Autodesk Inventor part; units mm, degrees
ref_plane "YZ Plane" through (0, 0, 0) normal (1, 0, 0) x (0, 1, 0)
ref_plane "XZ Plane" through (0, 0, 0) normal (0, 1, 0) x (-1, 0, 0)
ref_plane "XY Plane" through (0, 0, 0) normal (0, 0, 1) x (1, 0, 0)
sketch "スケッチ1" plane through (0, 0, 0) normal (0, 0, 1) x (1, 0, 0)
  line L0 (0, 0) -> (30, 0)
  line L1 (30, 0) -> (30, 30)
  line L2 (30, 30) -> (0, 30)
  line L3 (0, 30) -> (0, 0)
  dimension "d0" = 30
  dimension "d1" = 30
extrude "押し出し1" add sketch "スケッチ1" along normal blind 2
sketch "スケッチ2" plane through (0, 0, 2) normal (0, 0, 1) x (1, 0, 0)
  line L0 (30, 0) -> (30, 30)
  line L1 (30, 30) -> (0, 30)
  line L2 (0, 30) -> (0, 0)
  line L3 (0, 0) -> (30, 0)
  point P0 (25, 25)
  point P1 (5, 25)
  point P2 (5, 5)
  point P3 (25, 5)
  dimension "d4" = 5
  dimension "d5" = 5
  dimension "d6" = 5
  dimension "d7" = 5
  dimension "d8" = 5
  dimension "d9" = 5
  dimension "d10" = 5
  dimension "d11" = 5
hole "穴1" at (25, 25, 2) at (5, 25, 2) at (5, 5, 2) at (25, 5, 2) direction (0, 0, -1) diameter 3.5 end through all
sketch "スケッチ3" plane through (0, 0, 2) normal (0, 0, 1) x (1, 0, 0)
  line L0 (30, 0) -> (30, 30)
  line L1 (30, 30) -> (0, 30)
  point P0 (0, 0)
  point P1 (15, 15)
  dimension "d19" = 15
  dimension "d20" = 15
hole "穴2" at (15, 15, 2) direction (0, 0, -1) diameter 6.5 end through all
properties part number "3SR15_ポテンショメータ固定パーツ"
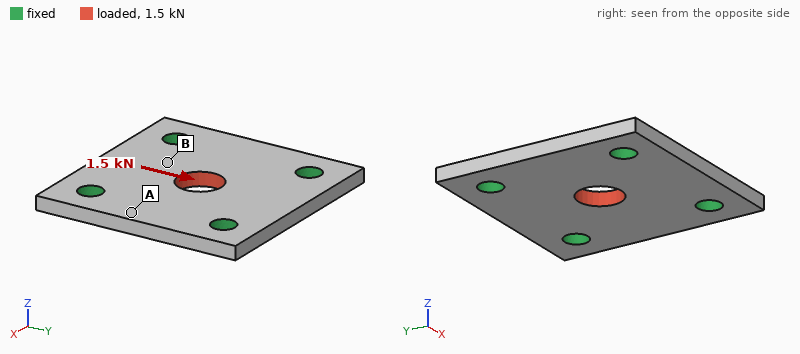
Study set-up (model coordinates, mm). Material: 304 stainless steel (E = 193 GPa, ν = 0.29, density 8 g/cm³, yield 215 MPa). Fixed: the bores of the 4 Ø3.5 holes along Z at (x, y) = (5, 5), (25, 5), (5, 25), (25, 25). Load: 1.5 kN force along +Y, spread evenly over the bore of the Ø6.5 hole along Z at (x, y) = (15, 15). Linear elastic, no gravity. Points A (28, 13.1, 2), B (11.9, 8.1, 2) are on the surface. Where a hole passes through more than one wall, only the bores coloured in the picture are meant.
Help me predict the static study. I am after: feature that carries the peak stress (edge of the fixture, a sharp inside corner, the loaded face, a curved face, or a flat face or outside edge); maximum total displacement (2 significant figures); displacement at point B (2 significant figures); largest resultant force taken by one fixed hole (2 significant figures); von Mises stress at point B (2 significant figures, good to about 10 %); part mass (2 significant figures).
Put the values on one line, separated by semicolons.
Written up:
edge of the fixture; 2.1 µm; 1.3 µm; 410 N; 24 MPa; 13 g
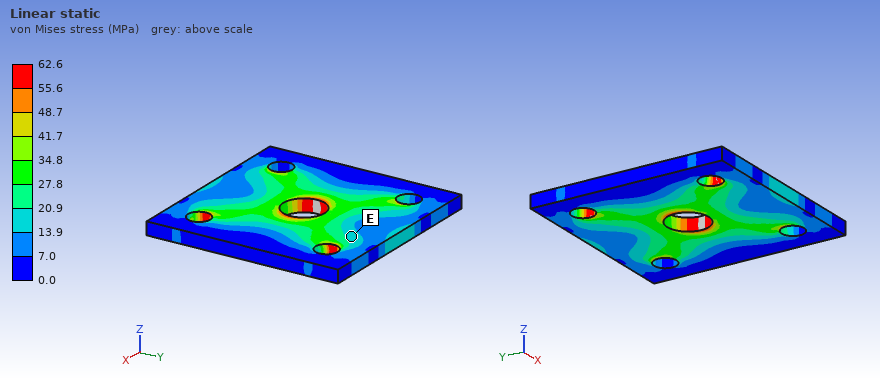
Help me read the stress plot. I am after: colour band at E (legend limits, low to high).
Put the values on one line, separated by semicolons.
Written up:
13.9 to 20.9 MPa
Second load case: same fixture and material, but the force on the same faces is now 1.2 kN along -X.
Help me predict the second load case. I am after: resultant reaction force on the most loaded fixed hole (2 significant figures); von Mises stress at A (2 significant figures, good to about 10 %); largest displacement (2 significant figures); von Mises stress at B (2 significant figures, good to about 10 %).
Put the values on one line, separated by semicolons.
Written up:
330 N; 8.3 MPa; 1.6 µm; 18 MPa
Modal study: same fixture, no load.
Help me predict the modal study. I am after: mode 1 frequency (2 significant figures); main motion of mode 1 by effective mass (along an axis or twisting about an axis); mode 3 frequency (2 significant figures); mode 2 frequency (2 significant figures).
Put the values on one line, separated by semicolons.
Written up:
22 kHz; along Z; 29 kHz; 29 kHz
